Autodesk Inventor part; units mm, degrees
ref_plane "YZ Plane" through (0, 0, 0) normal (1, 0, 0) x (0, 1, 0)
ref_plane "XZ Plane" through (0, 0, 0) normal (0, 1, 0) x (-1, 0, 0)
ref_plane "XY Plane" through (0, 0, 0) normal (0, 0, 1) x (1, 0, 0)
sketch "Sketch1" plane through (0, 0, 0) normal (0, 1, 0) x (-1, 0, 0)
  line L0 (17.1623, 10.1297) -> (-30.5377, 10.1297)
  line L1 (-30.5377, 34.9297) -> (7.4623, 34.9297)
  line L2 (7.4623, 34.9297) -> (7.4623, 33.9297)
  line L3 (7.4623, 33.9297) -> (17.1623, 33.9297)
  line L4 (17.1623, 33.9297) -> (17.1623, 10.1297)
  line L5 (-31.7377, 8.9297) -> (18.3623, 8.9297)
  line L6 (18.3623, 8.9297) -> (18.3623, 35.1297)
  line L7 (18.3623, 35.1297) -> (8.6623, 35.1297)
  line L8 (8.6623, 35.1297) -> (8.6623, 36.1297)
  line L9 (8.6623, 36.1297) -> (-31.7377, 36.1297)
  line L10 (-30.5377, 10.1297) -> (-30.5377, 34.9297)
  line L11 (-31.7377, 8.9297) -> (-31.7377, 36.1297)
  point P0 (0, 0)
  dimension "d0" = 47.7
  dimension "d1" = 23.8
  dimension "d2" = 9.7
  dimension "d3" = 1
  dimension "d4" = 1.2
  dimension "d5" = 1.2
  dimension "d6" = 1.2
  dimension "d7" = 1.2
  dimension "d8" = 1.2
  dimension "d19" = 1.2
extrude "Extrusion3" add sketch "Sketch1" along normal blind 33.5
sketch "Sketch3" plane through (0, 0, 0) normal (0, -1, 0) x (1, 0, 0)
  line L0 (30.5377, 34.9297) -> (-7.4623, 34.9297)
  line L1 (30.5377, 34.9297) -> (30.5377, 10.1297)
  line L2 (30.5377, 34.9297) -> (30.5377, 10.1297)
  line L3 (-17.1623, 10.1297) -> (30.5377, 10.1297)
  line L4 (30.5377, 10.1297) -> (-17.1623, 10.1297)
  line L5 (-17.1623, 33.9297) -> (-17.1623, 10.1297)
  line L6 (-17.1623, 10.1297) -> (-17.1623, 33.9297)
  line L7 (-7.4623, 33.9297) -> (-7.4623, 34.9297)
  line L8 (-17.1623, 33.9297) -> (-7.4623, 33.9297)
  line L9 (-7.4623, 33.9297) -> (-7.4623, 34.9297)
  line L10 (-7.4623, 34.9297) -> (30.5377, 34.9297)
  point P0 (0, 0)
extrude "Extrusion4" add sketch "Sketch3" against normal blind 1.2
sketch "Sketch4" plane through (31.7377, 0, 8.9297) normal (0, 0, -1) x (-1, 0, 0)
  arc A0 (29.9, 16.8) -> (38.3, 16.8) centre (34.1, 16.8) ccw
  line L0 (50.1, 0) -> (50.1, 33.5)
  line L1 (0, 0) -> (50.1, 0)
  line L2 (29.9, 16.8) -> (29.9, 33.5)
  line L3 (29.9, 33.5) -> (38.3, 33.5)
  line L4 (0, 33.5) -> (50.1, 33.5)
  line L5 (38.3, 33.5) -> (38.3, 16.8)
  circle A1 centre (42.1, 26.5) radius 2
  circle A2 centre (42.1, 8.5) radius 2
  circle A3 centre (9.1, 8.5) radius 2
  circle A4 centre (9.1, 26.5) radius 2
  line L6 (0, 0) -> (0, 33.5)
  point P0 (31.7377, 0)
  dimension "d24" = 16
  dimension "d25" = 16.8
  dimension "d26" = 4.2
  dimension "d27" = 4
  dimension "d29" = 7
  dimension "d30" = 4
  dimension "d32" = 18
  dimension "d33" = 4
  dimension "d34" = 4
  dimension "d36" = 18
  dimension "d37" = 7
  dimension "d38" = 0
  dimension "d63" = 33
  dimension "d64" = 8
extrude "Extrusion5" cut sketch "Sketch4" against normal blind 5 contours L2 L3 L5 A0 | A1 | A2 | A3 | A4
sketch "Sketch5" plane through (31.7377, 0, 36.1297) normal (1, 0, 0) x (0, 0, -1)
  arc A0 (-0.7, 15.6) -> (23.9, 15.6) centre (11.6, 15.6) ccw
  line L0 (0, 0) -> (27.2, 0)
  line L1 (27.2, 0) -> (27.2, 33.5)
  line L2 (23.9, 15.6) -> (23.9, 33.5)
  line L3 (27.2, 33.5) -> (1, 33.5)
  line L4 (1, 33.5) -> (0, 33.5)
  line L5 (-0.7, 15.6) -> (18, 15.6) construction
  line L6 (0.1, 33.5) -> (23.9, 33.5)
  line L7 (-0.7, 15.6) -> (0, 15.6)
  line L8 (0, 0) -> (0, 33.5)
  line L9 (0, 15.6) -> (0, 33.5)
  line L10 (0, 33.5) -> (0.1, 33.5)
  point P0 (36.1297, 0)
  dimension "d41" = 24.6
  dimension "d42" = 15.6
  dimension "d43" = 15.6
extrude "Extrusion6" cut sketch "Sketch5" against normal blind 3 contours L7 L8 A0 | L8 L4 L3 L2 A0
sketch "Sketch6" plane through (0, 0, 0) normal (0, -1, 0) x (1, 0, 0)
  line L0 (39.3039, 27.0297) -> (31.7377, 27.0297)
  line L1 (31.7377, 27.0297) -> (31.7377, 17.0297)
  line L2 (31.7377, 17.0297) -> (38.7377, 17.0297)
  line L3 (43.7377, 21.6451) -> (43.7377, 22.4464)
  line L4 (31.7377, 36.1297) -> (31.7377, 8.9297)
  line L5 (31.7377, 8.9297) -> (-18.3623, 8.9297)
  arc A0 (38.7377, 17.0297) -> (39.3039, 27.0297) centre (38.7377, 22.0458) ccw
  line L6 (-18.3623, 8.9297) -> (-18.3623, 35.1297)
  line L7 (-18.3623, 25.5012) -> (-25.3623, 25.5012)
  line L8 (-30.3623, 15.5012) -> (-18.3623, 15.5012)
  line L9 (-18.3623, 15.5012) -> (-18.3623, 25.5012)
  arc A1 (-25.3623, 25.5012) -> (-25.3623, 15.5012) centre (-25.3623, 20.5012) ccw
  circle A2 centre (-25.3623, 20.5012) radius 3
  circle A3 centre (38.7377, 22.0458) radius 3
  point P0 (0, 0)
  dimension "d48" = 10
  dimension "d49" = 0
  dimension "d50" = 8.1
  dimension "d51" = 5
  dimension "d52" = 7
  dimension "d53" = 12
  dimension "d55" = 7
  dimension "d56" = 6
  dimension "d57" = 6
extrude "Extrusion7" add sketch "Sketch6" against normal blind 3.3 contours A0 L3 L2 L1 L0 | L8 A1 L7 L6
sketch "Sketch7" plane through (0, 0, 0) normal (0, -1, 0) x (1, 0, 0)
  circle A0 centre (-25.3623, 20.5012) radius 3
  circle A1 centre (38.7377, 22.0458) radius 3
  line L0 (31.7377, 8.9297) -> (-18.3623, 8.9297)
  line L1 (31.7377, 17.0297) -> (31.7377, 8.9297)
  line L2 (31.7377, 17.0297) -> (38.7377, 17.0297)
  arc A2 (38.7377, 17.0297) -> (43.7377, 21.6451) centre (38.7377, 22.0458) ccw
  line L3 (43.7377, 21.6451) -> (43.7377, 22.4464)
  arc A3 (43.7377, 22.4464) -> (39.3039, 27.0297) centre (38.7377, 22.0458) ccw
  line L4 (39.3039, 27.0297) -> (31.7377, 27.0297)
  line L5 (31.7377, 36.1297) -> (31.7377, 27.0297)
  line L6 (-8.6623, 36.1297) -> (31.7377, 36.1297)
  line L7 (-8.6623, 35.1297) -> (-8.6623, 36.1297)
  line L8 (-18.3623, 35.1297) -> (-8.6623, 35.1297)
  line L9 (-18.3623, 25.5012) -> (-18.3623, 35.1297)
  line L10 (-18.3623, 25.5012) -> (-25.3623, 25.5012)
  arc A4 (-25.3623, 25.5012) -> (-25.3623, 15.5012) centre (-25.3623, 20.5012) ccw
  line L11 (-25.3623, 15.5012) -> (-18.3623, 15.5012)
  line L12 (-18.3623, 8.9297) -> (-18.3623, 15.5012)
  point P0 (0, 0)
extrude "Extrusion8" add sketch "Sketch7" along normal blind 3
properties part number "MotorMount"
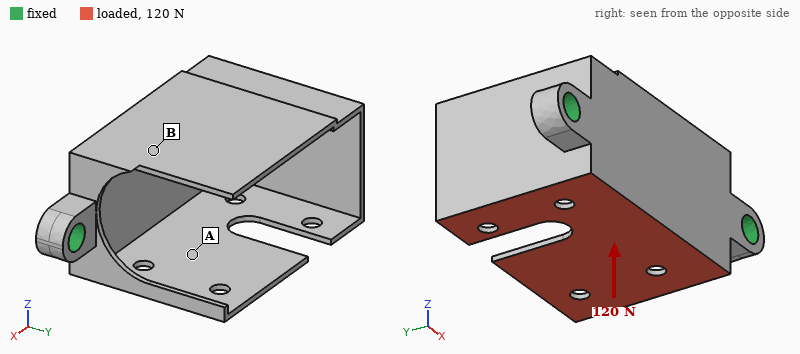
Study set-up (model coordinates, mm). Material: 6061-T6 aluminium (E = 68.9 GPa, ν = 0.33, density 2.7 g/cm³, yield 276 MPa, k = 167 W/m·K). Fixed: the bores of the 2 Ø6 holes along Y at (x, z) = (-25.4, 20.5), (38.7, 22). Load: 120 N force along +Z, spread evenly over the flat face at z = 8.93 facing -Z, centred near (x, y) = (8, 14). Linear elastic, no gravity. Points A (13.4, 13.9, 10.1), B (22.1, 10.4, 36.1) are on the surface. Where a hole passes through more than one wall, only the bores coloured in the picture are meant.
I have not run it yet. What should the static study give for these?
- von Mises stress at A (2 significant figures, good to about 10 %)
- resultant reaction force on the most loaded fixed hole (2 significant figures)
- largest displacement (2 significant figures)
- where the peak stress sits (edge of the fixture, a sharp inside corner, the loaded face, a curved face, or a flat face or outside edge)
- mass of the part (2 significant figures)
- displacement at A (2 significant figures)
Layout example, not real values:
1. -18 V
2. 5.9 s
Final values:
1. 26 MPa
2. 63 N
3. 0.46 mm
4. a curved face
5. 31 g
6. 0.10 mm
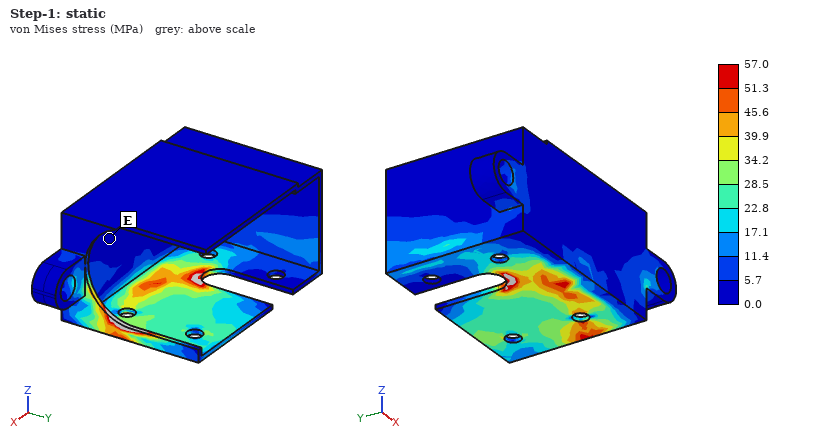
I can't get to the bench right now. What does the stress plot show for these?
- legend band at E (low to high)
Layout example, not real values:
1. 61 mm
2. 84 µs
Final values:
1. 0.0 to 5.7 MPa
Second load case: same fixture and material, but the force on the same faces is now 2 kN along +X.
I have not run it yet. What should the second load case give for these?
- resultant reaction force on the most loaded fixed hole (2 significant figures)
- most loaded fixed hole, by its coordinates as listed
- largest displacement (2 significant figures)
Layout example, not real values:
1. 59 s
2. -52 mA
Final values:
1. 1.3 kN
2. (-25.4, 20.5)
3. 0.32 mm
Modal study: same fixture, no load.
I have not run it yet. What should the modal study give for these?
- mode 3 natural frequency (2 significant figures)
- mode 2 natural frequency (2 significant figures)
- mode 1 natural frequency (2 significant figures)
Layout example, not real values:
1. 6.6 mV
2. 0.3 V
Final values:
1. 3400 Hz
2. 1600 Hz
3. 1500 Hz
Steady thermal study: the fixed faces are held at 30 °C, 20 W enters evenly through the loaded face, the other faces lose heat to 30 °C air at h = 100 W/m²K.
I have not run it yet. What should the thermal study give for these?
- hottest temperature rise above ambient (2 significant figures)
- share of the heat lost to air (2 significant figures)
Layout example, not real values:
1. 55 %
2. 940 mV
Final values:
1. 30 K
2. 39 %
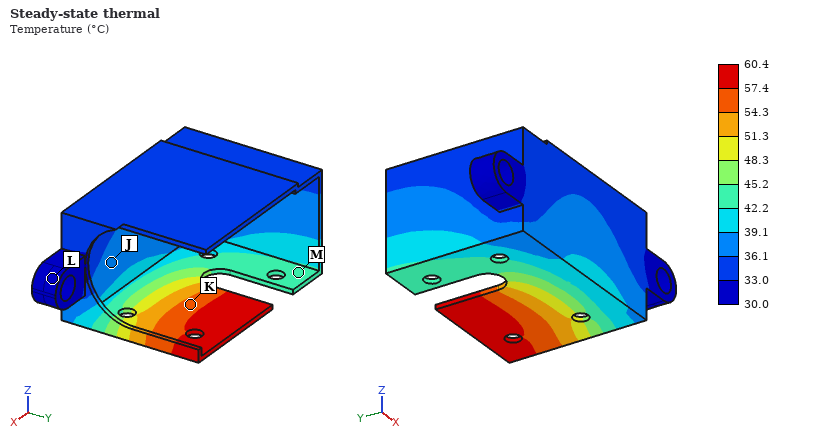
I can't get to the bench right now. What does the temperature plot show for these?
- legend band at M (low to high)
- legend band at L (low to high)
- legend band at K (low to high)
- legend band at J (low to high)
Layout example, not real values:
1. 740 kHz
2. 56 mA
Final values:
1. 42.2 to 45.2 °C
2. 30.0 to 33.0 °C
3. 54.3 to 57.4 °C
4. 36.1 to 39.1 °C
